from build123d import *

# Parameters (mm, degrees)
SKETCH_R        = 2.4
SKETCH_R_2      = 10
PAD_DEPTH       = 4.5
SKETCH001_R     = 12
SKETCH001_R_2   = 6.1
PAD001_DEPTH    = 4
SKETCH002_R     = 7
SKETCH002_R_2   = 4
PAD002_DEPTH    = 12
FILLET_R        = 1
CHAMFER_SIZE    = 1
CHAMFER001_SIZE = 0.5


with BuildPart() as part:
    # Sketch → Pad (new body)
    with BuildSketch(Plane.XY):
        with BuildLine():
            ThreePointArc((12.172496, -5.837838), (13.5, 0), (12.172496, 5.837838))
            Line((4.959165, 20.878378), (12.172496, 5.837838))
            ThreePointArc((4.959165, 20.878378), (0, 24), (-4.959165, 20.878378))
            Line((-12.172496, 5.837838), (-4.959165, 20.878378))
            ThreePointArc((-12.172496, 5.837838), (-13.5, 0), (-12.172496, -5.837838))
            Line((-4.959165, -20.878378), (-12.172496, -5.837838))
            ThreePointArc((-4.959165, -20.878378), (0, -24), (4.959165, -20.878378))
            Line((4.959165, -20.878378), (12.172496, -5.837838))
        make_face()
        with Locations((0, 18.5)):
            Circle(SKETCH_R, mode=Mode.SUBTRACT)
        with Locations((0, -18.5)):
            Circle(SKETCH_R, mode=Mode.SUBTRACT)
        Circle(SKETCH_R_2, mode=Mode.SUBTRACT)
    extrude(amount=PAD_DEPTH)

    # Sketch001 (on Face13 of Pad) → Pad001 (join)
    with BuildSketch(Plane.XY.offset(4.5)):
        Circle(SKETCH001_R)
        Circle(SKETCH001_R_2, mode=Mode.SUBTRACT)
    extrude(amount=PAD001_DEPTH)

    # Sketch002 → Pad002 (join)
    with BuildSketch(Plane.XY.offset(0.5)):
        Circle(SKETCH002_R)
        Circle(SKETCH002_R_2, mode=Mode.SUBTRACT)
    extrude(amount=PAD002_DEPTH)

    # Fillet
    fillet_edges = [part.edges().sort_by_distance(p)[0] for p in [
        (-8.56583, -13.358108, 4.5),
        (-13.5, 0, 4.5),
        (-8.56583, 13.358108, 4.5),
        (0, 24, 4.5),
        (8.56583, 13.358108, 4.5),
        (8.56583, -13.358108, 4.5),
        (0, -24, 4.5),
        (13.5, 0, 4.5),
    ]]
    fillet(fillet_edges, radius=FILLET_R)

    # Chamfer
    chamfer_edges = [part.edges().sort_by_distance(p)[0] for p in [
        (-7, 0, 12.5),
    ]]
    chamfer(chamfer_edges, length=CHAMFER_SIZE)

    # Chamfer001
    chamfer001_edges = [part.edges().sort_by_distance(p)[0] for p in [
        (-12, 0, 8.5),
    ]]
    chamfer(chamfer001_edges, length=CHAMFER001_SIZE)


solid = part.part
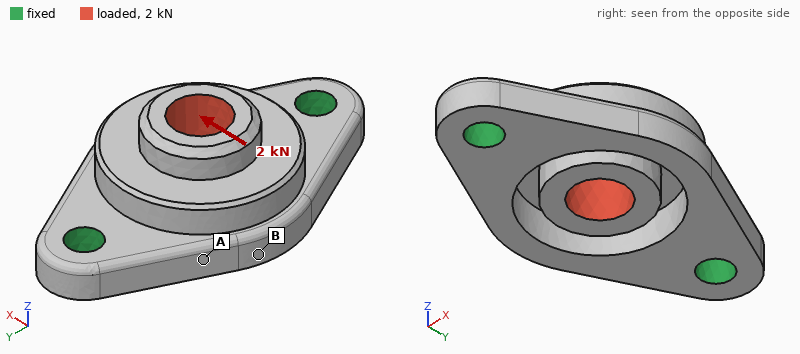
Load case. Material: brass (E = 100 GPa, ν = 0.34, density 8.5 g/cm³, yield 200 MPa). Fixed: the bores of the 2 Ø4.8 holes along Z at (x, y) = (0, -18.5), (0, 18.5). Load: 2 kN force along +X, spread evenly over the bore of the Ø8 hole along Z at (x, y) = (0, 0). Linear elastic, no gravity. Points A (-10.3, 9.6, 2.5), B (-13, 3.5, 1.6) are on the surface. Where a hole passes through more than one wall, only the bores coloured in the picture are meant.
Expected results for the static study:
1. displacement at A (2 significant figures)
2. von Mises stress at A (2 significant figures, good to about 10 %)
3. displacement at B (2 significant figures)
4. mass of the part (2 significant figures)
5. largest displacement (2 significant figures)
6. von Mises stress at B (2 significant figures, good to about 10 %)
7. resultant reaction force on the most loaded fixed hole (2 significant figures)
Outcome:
19 µm
44 MPa
27 µm
40 g
31 µm
14 MPa
1.0 kN
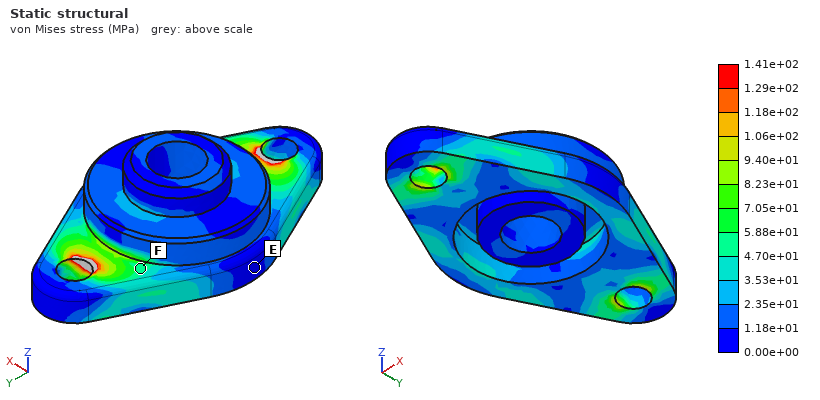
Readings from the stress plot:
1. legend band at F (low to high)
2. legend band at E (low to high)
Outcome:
4.70e+01 to 5.88e+01 MPa
0.00e+00 to 1.18e+01 MPa
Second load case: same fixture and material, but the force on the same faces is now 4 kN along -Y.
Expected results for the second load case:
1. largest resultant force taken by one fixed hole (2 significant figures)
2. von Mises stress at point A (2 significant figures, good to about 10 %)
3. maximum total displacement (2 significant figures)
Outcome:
2.1 kN
12 MPa
11 µm
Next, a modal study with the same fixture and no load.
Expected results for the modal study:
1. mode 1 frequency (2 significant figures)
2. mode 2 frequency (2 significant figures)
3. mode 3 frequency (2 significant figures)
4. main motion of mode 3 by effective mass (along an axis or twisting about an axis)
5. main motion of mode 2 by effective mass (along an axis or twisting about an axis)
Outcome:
7300 Hz
11 kHz
18 kHz
along X
along Z
